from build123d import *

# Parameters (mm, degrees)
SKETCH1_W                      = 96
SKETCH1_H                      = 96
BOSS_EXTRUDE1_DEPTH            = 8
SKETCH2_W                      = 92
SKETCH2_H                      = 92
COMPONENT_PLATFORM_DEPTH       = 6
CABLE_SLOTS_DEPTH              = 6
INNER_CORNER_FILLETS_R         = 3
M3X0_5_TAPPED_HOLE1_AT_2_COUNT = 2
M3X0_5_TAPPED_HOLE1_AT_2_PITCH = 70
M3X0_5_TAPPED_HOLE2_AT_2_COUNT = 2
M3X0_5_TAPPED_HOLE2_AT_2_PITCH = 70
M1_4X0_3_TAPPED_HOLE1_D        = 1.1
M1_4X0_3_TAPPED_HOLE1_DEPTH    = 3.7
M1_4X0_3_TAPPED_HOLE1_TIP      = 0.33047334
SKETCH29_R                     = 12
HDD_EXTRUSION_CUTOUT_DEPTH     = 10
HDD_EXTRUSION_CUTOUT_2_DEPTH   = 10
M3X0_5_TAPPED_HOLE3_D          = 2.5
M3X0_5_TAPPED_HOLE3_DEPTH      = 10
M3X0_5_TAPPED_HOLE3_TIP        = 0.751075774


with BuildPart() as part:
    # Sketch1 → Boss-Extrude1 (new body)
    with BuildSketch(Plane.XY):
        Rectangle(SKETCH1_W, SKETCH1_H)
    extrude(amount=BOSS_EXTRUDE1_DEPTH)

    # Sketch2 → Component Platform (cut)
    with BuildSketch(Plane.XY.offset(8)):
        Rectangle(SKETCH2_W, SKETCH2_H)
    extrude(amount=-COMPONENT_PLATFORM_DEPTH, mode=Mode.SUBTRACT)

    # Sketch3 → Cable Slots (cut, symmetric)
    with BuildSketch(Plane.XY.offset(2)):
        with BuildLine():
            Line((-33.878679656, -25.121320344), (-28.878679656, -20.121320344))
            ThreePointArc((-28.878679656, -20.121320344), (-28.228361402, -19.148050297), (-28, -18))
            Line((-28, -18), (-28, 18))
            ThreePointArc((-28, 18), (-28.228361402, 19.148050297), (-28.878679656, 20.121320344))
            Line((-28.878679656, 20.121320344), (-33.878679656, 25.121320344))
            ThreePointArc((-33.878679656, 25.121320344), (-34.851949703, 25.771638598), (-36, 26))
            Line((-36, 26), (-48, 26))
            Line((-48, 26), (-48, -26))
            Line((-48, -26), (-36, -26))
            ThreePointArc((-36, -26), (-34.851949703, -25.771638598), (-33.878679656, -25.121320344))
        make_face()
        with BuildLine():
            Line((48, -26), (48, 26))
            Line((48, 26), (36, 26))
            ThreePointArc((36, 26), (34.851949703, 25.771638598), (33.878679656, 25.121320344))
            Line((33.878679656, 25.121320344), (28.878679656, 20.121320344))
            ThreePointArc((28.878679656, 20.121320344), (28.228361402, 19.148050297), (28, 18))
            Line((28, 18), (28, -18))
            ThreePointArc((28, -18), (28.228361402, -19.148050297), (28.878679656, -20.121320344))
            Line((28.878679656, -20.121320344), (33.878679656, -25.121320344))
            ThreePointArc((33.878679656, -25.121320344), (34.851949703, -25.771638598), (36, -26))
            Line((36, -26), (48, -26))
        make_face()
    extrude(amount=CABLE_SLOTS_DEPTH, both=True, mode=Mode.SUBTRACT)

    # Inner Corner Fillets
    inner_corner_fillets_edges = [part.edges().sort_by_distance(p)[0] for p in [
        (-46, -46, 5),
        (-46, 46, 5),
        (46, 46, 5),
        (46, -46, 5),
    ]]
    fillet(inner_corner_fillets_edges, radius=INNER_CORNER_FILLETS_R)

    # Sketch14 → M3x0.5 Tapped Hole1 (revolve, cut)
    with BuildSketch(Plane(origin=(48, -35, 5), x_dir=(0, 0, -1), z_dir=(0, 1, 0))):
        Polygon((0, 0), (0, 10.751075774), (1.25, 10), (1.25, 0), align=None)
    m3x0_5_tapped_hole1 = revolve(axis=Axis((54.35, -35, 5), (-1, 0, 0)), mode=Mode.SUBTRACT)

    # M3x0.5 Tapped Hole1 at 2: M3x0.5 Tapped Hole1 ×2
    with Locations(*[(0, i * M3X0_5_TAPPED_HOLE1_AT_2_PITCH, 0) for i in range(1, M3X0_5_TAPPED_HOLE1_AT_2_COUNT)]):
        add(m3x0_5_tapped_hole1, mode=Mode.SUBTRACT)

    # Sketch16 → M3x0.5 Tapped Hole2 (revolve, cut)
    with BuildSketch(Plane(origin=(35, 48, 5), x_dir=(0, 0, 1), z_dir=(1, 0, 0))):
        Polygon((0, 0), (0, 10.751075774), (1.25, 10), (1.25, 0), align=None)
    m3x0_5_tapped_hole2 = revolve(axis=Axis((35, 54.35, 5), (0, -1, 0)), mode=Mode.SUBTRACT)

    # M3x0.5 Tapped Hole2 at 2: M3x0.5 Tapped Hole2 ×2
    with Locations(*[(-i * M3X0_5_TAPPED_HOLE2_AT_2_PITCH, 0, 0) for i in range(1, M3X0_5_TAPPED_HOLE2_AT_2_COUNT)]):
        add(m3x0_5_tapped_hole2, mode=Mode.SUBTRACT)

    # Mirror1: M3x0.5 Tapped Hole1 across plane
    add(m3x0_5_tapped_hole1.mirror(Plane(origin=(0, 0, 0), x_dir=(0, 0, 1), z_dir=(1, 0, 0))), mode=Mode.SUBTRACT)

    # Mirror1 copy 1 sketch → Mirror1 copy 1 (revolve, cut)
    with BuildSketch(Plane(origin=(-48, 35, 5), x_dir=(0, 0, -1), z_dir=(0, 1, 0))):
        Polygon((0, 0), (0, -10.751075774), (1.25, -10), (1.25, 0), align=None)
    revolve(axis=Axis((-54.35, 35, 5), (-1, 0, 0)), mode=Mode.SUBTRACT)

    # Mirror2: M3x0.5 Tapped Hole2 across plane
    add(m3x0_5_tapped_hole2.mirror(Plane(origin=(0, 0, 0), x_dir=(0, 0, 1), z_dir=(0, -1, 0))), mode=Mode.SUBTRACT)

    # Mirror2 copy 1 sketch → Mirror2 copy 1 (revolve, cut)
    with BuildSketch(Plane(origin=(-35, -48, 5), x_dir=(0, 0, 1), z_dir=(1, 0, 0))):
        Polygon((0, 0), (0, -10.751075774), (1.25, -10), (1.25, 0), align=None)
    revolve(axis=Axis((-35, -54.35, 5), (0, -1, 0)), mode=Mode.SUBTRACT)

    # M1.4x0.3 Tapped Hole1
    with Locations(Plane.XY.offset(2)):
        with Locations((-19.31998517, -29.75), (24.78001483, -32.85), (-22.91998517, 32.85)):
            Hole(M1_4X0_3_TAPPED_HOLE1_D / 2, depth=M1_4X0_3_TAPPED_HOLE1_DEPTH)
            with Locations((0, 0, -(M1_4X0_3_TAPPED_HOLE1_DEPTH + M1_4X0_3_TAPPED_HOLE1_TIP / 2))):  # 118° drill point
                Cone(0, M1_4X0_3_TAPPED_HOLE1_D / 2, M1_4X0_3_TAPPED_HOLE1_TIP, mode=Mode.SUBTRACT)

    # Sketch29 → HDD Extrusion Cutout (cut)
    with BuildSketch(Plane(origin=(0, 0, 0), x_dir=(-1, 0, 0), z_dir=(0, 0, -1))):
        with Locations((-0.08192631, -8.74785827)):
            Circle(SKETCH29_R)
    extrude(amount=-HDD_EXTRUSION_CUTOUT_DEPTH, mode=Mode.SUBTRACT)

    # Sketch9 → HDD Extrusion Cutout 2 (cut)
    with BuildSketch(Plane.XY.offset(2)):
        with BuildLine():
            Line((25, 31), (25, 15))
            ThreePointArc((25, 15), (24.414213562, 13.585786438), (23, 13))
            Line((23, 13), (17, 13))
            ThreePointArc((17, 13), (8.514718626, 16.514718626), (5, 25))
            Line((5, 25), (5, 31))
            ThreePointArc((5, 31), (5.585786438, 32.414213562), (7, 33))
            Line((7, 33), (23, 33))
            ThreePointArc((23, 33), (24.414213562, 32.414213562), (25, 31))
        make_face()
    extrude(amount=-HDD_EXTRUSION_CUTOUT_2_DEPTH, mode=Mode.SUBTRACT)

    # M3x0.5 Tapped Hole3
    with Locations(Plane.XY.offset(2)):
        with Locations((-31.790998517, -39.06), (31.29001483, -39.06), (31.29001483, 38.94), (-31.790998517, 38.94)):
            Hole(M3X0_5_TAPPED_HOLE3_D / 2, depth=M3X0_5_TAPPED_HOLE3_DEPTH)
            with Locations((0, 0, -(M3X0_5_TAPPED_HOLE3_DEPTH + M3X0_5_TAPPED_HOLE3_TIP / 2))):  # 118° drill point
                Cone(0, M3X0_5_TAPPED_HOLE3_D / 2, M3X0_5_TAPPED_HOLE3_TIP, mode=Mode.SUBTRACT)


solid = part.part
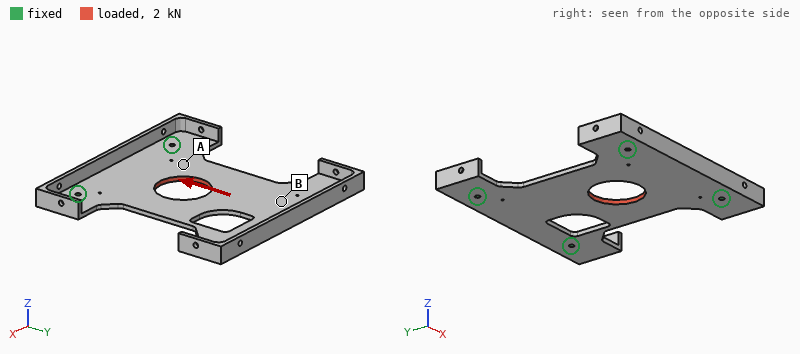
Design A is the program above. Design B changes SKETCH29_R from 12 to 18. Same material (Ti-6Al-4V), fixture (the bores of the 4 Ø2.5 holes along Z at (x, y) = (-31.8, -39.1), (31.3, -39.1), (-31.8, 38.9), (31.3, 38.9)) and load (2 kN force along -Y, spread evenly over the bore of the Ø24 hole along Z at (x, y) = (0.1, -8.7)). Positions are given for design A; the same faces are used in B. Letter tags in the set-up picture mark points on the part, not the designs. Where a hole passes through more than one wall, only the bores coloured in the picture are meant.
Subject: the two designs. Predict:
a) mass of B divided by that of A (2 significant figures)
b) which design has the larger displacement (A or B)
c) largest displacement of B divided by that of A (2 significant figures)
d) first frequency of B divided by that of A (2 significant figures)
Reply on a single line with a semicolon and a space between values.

0.93; B; 1.3; 1.1
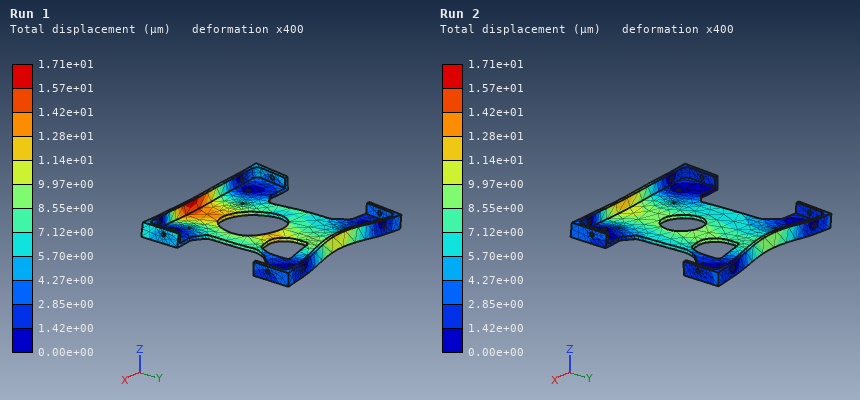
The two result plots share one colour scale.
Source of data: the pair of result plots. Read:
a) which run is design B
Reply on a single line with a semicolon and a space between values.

Run 1
